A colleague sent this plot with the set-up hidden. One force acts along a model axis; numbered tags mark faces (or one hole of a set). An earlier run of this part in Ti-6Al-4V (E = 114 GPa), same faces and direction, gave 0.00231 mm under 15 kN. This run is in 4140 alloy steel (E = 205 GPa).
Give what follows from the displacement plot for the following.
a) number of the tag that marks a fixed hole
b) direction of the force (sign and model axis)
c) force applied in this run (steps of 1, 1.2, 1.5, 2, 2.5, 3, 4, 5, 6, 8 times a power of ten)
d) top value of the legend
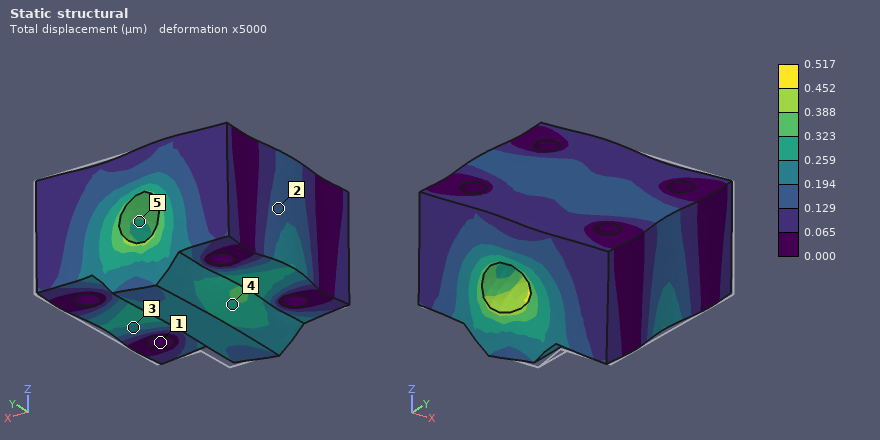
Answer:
1
-X
6 kN
0.517 µm
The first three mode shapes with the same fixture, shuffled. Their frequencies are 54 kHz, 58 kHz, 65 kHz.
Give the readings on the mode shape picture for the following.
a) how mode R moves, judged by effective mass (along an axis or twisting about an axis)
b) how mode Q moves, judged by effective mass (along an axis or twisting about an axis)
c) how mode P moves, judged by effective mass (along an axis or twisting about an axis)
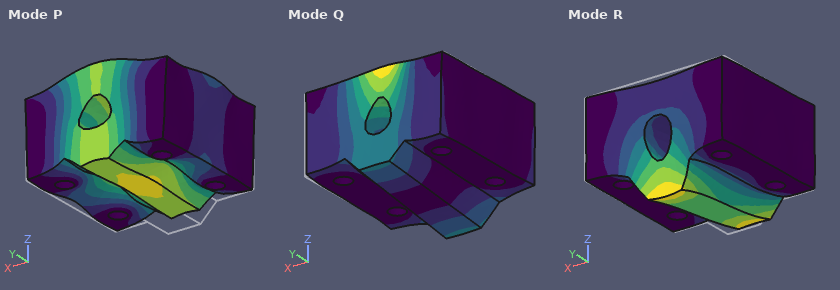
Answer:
along Y
along Y
along Z
